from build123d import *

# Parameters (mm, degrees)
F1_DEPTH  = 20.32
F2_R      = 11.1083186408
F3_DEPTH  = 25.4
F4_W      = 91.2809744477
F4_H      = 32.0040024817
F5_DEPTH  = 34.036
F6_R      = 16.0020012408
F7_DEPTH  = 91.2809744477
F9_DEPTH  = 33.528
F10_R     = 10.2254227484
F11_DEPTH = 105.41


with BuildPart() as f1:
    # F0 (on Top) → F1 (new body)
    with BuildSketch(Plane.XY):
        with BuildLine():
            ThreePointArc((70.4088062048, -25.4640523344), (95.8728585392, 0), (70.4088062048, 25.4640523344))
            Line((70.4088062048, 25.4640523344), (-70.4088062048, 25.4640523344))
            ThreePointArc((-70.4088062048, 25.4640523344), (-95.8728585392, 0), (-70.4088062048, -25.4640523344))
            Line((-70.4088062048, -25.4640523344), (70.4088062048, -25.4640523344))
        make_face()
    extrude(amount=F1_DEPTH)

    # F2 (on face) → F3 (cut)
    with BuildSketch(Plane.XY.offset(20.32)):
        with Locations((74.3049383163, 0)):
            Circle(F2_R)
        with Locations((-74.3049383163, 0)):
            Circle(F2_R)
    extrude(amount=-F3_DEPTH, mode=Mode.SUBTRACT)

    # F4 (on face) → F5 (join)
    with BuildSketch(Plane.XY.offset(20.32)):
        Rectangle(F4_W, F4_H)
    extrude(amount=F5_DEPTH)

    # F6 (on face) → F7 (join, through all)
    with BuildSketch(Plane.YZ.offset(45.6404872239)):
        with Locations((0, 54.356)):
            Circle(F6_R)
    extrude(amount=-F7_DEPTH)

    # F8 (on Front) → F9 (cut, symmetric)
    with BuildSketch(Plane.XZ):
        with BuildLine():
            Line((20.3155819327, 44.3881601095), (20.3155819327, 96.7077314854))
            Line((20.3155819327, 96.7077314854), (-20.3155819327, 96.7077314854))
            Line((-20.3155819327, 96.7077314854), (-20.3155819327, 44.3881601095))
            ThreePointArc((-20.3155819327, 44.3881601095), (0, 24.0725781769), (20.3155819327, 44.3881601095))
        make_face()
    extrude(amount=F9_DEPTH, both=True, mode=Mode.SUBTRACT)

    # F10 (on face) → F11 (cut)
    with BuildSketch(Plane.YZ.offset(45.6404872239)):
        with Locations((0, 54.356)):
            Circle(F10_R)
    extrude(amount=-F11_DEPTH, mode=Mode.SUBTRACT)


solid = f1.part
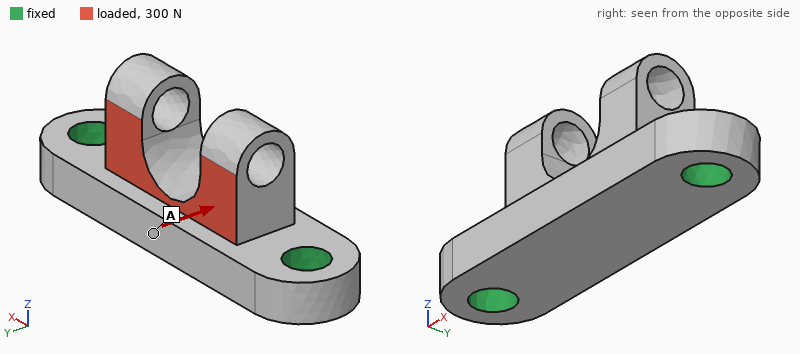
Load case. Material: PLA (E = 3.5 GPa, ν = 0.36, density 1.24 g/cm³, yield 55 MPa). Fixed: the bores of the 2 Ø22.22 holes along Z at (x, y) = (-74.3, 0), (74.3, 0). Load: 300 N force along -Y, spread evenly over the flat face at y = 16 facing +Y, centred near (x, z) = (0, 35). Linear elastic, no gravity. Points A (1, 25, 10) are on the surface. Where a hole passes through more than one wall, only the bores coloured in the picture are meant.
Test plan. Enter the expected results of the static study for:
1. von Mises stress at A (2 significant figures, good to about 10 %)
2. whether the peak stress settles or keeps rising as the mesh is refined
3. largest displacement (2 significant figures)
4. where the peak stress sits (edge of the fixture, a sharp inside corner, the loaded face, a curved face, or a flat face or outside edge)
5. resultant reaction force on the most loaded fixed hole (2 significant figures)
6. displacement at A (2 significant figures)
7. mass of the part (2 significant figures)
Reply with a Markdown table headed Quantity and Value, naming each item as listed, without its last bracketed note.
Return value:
| Quantity | Value |
|---|---|
| von Mises stress at A | 0.27 MPa |
| whether the peak stress settles or keeps rising as the mesh is refined | keeps rising |
| largest displacement | 55 µm |
| where the peak stress sits | edge of the fixture |
| resultant reaction force on the most loaded fixed hole | 150 N |
| displacement at A | 20 µm |
| mass of the part | 300 g |
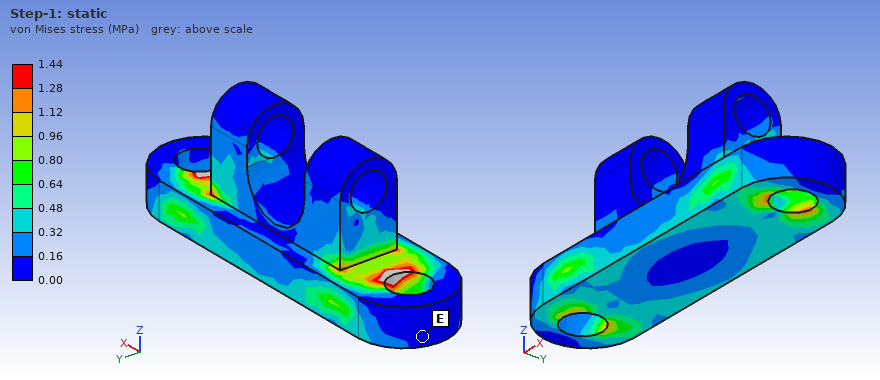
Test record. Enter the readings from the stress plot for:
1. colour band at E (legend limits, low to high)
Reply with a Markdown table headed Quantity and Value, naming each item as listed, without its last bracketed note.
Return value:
| Quantity | Value |
|---|---|
| colour band at E | 0.00 to 0.16 MPa |
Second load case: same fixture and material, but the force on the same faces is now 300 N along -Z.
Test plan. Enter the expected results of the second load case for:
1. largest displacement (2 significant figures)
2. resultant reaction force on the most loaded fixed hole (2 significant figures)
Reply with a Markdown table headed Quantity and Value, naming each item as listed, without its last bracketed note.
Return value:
| Quantity | Value |
|---|---|
| largest displacement | 40 µm |
| resultant reaction force on the most loaded fixed hole | 160 N |
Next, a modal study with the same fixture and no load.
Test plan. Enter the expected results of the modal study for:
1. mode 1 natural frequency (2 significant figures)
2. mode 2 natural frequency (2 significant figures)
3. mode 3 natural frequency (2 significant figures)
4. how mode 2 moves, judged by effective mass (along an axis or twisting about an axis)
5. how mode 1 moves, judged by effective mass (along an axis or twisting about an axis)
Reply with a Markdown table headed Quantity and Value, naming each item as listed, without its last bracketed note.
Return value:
| Quantity | Value |
|---|---|
| mode 1 natural frequency | 1300 Hz |
| mode 2 natural frequency | 1400 Hz |
| mode 3 natural frequency | 2100 Hz |
| how mode 2 moves, judged by effective mass | along Z |
| how mode 1 moves, judged by effective mass | along Y |
